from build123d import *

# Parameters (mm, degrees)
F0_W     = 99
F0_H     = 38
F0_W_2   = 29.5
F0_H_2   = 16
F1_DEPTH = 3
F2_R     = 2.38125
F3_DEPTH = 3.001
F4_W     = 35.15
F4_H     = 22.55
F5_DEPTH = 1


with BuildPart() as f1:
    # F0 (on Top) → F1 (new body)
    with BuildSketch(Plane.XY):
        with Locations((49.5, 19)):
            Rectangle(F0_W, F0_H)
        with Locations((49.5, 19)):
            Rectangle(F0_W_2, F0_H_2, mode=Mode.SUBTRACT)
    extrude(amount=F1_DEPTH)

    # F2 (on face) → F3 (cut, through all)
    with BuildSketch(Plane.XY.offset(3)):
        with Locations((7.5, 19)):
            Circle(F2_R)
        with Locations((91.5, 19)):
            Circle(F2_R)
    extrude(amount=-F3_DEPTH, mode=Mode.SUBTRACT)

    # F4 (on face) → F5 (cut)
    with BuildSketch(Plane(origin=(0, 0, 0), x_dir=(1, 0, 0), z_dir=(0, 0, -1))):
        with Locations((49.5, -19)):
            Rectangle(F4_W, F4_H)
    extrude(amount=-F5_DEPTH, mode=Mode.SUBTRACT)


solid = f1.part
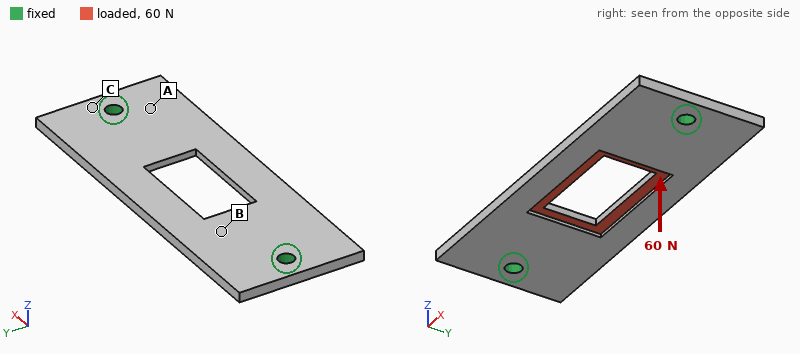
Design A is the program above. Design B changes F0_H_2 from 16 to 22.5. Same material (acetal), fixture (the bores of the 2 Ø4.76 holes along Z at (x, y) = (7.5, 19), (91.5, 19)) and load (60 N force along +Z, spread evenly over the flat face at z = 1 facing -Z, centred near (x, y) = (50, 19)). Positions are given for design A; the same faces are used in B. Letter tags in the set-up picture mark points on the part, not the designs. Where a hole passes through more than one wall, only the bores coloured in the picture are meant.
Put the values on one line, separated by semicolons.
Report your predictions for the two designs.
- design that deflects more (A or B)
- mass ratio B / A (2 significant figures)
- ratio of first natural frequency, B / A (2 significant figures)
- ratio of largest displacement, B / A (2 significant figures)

A; 0.96; 1.0; 0.80
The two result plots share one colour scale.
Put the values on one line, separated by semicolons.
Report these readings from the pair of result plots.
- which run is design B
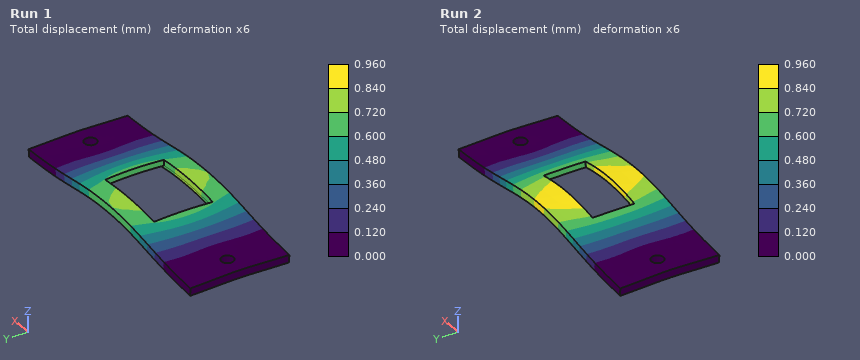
Run 1
